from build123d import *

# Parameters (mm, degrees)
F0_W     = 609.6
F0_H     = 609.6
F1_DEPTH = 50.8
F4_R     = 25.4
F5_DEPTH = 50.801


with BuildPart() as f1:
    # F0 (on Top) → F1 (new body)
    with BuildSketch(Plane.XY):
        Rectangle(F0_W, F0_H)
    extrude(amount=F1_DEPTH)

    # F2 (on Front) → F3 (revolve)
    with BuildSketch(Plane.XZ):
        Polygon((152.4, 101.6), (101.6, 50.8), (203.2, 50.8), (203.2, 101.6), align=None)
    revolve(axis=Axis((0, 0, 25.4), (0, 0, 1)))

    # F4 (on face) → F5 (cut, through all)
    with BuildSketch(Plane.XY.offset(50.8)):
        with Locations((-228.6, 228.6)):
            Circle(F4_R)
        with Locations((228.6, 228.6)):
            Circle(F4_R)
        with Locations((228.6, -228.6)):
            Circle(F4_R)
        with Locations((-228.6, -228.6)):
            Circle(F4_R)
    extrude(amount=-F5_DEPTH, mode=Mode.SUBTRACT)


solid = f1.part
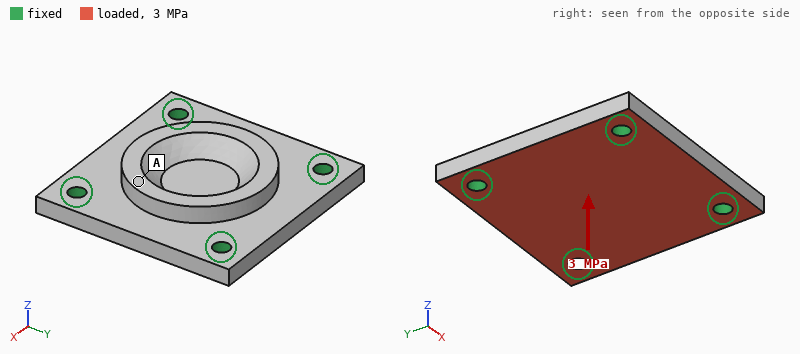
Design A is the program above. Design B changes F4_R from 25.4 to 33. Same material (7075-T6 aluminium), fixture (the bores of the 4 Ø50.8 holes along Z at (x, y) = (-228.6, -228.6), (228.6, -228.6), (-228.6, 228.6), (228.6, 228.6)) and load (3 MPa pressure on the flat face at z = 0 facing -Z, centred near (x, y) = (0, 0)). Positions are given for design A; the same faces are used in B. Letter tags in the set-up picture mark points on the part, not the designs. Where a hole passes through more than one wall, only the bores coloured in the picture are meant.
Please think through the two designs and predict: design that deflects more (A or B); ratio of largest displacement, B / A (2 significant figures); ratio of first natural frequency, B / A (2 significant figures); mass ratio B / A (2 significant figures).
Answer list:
A
0.86
1.1
0.99
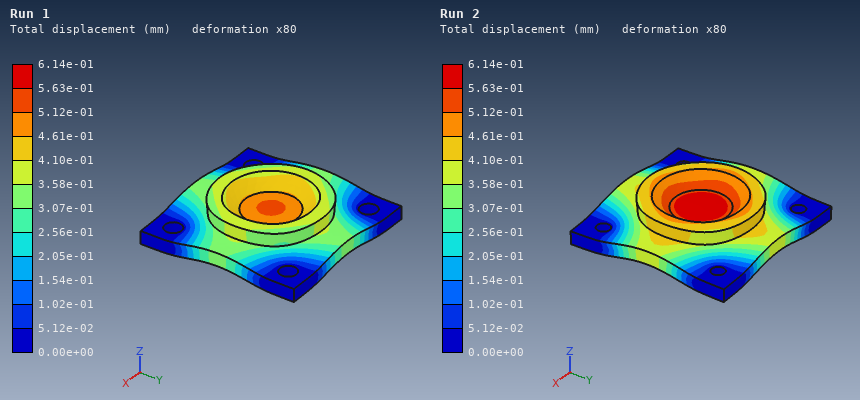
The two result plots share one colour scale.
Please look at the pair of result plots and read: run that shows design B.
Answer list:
Run 1
